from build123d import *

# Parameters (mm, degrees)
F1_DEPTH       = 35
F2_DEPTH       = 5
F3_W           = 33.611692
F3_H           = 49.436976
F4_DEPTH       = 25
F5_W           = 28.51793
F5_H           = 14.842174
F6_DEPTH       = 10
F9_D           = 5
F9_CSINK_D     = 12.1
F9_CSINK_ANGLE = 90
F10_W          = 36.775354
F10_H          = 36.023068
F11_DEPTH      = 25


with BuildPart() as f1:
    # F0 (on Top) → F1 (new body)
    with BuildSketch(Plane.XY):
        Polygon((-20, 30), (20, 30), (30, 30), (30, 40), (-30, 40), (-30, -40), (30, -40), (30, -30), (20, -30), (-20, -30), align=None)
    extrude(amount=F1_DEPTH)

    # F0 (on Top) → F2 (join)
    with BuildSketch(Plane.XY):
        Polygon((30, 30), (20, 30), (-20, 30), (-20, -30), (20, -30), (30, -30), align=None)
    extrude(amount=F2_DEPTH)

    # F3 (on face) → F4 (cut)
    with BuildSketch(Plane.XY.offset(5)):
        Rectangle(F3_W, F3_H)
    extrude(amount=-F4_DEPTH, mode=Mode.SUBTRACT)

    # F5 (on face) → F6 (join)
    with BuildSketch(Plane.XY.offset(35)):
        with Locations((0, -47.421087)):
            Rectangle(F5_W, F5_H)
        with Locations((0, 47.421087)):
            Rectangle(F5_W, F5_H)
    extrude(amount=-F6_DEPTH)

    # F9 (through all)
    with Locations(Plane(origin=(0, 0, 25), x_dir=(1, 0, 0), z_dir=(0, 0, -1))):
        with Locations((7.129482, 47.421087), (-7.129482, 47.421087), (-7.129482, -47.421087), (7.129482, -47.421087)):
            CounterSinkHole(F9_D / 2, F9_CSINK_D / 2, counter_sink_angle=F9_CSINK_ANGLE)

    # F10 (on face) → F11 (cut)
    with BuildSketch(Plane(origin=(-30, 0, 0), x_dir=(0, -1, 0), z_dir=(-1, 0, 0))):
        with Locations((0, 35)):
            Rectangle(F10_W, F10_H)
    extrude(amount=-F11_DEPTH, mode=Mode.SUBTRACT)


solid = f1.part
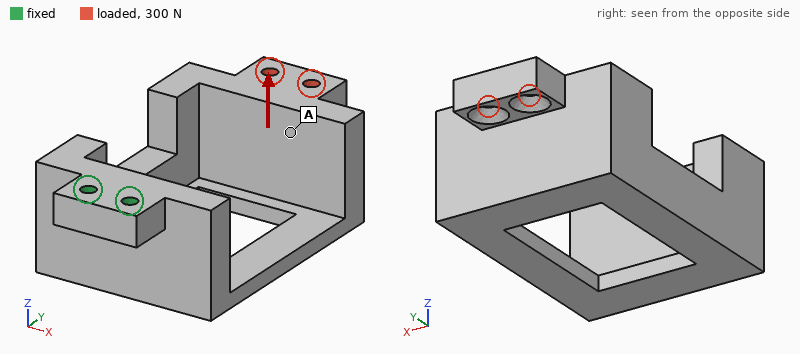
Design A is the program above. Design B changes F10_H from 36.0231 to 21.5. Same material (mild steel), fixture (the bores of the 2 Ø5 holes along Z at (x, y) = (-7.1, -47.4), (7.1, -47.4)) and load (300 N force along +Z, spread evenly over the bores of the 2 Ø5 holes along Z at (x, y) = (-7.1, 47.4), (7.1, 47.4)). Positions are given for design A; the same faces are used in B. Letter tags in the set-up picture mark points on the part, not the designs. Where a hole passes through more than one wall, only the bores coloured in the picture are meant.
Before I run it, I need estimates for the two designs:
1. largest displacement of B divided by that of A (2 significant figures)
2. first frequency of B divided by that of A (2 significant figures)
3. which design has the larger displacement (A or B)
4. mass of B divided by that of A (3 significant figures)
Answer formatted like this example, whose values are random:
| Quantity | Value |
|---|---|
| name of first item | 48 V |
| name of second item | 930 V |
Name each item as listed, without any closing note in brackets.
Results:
| Quantity | Value |
|---|---|
| largest displacement of B divided by that of A | 0.82 |
| first frequency of B divided by that of A | 1.1 |
| which design has the larger displacement | A |
| mass of B divided by that of A | 1.04 |
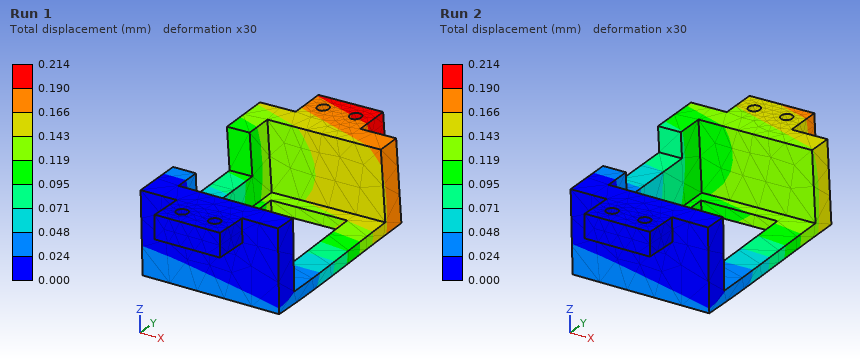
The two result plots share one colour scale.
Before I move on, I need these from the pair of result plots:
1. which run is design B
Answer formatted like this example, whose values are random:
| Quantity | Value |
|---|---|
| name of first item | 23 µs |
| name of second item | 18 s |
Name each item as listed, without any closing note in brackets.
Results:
| Quantity | Value |
|---|---|
| which run is design B | Run 2 |
